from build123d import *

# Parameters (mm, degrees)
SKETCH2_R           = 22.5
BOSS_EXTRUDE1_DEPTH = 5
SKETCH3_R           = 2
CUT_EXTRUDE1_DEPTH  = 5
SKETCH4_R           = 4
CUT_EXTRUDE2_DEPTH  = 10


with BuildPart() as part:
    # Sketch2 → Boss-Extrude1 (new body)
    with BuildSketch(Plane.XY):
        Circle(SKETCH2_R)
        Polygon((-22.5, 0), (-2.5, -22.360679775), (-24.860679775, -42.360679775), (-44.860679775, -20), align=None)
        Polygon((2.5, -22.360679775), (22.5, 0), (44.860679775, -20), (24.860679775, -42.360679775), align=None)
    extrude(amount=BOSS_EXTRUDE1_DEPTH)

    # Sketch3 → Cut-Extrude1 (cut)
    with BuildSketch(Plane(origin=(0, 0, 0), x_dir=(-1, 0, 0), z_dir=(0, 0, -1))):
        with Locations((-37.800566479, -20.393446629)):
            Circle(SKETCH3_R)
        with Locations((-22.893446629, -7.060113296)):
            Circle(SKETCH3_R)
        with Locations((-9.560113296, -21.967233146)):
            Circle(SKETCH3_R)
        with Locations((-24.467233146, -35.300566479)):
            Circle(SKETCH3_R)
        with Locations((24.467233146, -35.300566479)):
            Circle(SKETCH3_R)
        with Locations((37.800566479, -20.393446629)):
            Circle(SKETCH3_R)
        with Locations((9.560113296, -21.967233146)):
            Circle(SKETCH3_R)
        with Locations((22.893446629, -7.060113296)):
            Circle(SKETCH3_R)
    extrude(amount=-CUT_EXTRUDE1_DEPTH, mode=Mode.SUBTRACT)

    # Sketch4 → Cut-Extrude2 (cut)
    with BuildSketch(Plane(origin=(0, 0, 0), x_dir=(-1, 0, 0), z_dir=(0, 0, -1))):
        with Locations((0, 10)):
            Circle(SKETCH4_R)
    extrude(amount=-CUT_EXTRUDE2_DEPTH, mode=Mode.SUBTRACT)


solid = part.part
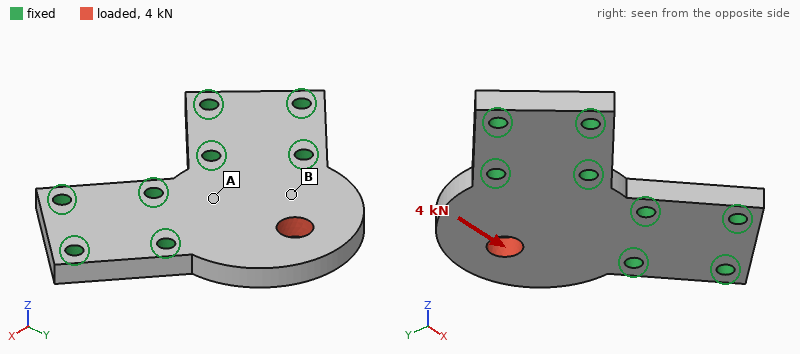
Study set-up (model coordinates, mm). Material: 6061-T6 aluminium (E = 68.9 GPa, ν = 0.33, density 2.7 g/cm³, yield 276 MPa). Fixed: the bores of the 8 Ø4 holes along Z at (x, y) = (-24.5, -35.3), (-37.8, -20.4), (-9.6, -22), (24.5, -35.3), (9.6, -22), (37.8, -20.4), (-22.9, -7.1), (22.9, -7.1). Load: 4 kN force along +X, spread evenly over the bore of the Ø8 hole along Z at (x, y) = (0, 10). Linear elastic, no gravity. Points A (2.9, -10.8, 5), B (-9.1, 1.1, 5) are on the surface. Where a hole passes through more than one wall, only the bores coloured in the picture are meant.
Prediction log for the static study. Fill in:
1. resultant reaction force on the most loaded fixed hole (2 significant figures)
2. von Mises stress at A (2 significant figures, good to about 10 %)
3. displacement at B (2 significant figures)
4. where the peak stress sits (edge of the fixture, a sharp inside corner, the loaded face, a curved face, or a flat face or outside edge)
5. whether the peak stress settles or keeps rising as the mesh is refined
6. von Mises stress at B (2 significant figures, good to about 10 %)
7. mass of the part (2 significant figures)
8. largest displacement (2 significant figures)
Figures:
2.1 kN
11 MPa
7.6 µm
edge of the fixture
keeps rising
30 MPa
41 g
22 µm
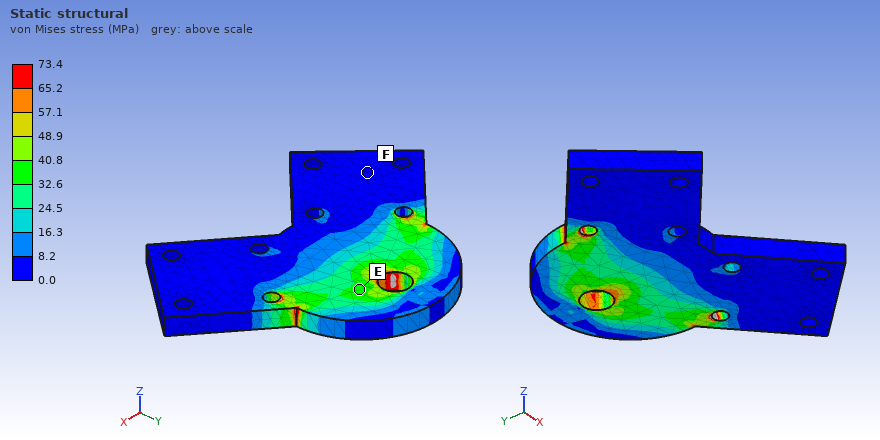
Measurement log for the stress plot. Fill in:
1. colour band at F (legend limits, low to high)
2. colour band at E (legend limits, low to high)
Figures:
0.0 to 8.2 MPa
32.6 to 40.8 MPa
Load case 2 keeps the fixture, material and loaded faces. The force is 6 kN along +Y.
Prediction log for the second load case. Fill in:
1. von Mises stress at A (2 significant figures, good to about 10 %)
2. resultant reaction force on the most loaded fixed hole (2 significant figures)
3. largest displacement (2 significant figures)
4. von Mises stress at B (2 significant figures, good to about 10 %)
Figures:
23 MPa
1.6 kN
21 µm
34 MPa
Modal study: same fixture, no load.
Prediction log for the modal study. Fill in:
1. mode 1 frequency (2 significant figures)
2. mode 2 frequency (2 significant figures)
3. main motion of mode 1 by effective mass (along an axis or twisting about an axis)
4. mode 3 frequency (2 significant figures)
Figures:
4700 Hz
12 kHz
along Z
18 kHz
